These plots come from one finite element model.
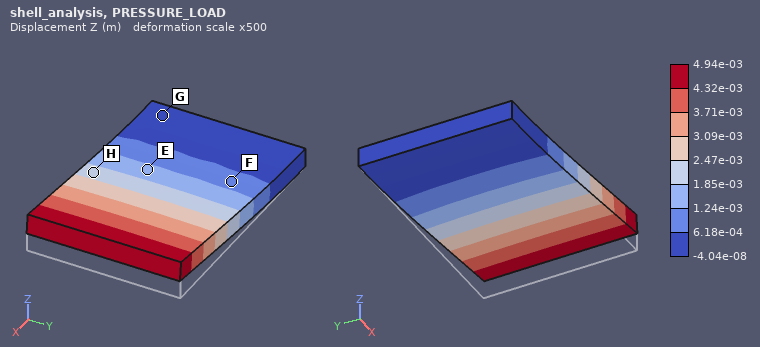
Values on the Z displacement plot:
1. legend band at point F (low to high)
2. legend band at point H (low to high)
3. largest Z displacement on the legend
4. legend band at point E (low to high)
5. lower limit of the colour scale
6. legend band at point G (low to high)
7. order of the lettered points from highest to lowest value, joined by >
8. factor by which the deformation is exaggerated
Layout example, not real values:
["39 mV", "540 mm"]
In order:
["6.18e-04 to 1.24e-03 m", "1.85e-03 to 2.47e-03 m", "4.94e-03 m", "1.24e-03 to 1.85e-03 m", "-4.04e-08 m", "-4.04e-08 to 6.18e-04 m", "H > E > F > G", "500"]
